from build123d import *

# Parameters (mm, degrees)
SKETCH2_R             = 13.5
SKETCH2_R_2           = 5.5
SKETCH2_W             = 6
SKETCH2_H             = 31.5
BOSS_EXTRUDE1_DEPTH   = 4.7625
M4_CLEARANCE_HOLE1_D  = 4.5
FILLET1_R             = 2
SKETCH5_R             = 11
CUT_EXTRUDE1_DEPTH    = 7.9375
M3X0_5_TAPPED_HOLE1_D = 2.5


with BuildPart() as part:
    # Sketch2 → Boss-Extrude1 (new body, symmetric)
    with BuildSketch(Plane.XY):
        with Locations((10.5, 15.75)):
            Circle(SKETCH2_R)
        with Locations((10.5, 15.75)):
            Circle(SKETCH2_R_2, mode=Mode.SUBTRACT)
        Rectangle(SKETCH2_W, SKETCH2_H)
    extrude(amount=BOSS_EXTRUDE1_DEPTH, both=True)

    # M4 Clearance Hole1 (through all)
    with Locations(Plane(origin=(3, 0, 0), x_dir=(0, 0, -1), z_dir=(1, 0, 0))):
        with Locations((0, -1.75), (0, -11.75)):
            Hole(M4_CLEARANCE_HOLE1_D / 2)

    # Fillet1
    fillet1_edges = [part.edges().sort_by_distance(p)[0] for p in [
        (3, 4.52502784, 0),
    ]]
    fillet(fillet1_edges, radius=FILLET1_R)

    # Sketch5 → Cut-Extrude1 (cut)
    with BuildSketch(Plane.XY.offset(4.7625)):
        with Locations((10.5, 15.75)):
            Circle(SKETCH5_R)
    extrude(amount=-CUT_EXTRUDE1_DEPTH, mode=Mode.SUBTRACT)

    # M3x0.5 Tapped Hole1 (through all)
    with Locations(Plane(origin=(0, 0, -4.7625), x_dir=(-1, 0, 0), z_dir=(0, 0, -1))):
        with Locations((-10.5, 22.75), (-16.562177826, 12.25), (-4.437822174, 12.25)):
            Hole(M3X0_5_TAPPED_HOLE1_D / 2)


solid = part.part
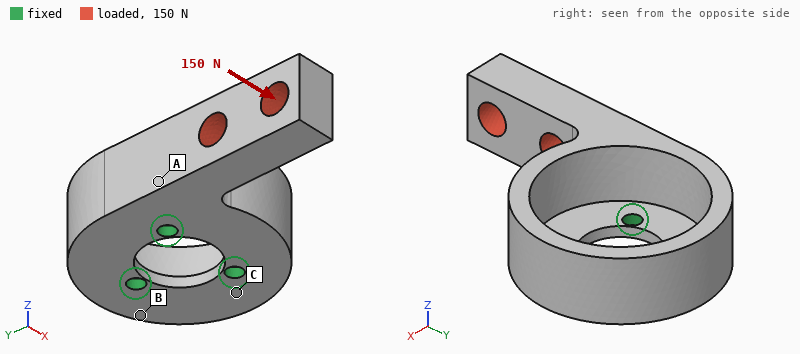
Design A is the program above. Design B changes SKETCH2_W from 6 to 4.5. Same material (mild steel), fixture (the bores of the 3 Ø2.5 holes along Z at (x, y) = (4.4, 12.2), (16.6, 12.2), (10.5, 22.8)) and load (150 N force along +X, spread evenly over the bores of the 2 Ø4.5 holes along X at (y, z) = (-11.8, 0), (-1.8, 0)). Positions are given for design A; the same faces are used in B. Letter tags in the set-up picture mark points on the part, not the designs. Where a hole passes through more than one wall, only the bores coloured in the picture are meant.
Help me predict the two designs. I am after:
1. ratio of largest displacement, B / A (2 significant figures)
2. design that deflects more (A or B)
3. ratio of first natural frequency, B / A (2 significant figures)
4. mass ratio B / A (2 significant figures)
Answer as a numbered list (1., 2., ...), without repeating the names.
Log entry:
1. 1.7
2. B
3. 1.1
4. 0.91
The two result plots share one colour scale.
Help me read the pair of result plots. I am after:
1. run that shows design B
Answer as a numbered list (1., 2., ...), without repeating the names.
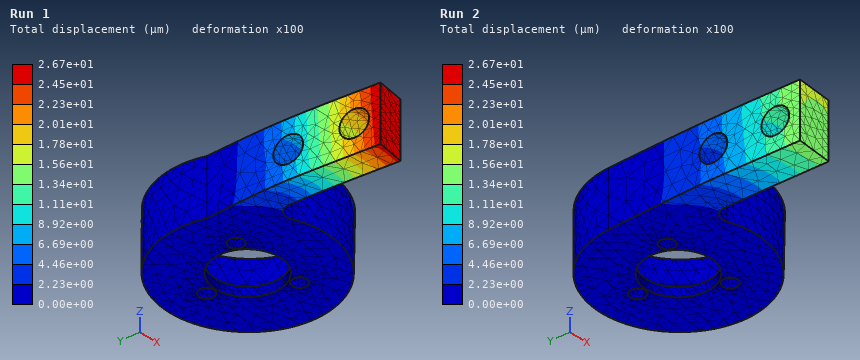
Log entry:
1. Run 1
